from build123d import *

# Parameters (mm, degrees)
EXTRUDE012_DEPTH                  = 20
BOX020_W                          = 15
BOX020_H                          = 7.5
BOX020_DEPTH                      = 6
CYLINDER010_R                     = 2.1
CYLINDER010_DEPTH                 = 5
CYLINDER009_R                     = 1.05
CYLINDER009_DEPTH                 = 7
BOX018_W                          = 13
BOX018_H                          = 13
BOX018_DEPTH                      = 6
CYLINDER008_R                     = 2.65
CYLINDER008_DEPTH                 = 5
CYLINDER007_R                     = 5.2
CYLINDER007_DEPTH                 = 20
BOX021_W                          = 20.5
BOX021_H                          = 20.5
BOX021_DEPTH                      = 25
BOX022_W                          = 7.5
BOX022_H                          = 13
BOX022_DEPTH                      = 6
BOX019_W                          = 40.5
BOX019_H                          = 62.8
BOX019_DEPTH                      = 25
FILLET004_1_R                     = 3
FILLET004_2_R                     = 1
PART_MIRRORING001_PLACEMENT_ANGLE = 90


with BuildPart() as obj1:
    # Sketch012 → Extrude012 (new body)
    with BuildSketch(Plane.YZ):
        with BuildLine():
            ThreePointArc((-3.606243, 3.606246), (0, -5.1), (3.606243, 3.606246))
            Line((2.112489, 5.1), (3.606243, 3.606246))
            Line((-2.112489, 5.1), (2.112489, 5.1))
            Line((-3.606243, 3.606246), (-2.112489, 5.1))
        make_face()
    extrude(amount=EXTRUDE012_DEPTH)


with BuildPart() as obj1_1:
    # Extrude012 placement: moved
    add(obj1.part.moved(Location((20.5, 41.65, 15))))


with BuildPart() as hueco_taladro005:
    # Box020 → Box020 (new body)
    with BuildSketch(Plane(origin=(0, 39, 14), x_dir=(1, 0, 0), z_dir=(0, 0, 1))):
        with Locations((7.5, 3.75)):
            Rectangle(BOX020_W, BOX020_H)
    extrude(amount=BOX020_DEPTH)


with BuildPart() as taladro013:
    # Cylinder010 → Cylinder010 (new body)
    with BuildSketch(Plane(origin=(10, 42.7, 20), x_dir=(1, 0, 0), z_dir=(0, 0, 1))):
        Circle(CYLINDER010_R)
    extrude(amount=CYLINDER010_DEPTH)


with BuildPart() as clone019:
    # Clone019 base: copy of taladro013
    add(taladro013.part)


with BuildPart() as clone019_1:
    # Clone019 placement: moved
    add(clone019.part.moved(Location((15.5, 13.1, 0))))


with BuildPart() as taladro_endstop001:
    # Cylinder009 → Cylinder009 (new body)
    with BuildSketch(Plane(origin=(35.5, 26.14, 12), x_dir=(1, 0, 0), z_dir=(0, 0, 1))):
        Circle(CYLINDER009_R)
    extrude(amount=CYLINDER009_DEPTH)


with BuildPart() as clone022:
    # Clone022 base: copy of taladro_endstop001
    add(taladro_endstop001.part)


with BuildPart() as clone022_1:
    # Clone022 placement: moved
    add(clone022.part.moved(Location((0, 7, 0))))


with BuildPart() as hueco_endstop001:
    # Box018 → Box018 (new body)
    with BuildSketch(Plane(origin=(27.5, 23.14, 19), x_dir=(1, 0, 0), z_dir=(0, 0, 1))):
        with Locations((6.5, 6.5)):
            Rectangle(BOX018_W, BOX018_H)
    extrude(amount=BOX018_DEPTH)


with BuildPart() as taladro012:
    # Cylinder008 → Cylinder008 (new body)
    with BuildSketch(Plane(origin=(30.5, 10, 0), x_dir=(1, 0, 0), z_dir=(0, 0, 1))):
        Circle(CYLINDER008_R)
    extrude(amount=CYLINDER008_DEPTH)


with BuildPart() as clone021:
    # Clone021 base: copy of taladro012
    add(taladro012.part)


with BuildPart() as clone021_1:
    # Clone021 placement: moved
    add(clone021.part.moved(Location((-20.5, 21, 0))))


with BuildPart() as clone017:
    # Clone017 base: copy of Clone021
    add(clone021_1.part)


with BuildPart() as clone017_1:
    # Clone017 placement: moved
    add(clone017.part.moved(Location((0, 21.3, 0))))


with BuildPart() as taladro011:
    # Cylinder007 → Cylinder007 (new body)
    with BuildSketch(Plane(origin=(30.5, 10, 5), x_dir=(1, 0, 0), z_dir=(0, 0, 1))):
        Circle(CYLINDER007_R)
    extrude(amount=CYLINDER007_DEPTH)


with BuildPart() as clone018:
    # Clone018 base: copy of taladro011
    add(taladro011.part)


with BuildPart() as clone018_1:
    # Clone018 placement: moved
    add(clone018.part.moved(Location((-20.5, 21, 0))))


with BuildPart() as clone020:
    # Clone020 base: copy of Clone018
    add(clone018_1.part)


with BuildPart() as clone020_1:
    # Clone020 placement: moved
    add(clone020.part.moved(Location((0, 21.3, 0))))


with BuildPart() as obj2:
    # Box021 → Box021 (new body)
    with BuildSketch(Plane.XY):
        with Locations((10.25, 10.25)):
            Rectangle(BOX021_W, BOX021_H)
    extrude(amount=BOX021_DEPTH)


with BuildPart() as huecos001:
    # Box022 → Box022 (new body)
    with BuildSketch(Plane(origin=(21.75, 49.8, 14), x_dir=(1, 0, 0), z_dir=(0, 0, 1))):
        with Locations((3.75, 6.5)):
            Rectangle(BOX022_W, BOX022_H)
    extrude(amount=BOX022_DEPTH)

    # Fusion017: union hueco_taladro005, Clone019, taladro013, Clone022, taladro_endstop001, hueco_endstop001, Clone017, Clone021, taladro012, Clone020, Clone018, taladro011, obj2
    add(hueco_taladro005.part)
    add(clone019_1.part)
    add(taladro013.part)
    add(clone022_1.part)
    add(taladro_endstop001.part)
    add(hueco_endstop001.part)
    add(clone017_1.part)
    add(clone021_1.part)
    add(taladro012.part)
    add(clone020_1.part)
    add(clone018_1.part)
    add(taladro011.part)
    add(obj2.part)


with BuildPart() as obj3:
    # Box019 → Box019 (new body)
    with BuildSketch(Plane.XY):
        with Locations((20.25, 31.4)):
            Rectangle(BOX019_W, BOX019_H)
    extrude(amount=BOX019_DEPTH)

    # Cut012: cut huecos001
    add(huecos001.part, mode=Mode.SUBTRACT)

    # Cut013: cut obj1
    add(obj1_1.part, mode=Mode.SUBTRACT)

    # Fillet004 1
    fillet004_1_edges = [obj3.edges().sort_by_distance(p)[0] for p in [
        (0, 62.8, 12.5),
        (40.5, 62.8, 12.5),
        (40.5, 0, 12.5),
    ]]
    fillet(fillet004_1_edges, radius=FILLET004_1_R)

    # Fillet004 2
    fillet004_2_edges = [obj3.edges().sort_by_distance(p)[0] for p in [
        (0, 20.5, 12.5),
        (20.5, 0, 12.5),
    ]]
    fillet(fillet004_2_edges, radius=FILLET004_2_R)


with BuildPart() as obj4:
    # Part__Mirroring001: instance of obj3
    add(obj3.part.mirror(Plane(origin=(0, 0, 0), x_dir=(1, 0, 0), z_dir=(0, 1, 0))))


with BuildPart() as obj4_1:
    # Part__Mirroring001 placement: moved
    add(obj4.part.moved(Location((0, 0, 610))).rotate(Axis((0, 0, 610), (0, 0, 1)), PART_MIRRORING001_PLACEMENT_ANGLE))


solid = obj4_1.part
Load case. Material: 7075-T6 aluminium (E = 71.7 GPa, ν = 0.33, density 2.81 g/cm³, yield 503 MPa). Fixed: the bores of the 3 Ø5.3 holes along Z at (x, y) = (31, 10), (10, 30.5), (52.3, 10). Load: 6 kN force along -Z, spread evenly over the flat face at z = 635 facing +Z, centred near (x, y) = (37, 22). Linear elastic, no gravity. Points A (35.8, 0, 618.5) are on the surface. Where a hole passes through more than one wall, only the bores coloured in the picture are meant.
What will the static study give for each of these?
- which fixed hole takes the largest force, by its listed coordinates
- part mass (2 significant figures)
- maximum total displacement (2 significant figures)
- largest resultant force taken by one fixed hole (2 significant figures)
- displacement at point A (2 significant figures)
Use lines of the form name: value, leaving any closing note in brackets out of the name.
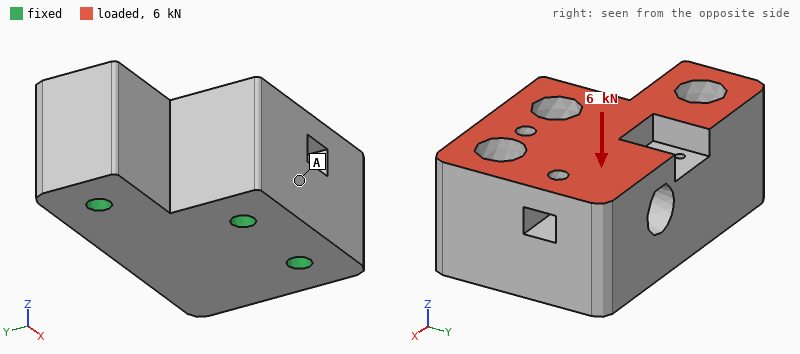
which fixed hole takes the largest force, by its listed coordinates: (52.3, 10)
part mass: 120 g
maximum total displacement: 50 µm
largest resultant force taken by one fixed hole: 3.5 kN
displacement at point A: 7.9 µm
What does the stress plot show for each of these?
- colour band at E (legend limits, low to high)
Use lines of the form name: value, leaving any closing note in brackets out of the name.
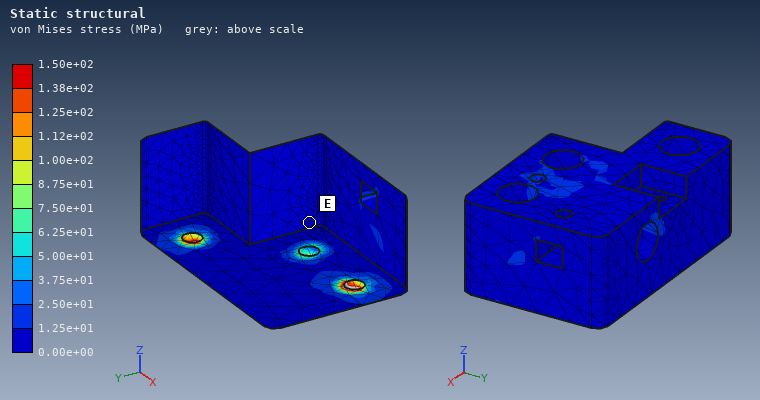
colour band at E: 0.00e+00 to 1.25e+01 MPa
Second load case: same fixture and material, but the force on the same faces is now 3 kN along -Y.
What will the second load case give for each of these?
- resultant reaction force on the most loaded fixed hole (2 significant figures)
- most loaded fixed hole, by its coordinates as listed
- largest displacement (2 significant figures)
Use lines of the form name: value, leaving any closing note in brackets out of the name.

resultant reaction force on the most loaded fixed hole: 3.1 kN
most loaded fixed hole, by its coordinates as listed: (31, 10)
largest displacement: 61 µm
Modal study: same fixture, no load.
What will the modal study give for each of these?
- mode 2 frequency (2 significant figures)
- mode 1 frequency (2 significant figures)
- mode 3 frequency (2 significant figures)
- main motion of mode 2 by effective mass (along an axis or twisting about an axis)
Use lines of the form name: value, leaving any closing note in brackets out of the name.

mode 2 frequency: 14 kHz
mode 1 frequency: 5200 Hz
mode 3 frequency: 14 kHz
main motion of mode 2 by effective mass: along X
